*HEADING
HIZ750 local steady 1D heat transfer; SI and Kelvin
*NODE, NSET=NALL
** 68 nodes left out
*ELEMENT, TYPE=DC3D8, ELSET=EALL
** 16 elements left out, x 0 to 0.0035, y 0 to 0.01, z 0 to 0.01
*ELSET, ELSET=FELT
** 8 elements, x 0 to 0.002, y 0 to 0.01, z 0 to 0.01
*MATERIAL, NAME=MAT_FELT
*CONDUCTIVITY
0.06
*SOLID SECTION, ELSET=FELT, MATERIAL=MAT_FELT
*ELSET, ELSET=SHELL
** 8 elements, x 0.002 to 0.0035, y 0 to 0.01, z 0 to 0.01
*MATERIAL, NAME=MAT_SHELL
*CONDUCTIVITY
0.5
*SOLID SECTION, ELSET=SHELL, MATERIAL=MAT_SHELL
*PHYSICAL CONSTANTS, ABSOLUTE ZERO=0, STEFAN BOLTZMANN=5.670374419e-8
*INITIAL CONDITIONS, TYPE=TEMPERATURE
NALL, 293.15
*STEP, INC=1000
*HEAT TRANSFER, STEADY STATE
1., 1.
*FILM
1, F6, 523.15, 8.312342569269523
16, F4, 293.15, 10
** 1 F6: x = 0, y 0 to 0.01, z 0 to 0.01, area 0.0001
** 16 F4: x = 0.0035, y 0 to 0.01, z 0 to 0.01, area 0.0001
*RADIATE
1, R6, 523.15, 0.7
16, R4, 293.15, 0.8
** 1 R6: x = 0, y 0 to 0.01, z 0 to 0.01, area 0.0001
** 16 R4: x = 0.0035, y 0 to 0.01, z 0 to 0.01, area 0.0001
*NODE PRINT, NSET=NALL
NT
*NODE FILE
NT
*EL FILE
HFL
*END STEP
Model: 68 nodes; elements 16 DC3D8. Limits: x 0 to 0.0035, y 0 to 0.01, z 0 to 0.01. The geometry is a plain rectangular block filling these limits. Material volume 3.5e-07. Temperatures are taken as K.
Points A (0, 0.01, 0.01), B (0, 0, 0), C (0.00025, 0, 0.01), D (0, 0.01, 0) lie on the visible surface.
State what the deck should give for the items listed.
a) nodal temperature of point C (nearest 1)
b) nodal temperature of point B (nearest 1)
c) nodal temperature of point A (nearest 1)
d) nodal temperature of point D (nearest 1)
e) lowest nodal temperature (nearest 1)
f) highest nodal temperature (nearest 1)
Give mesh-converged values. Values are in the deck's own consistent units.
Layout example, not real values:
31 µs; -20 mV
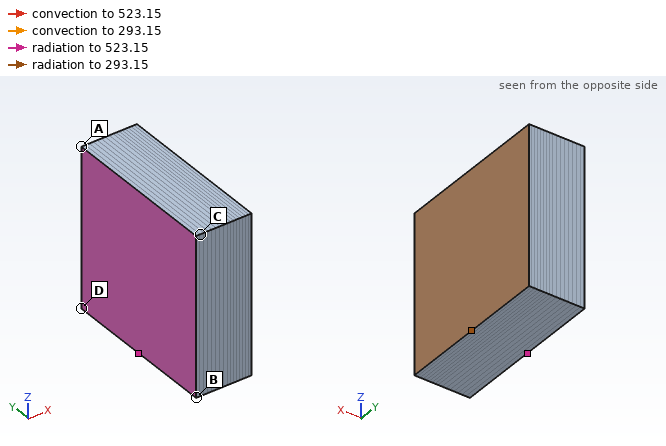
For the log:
451 K; 458 K; 458 K; 458 K; 394 K; 458 K
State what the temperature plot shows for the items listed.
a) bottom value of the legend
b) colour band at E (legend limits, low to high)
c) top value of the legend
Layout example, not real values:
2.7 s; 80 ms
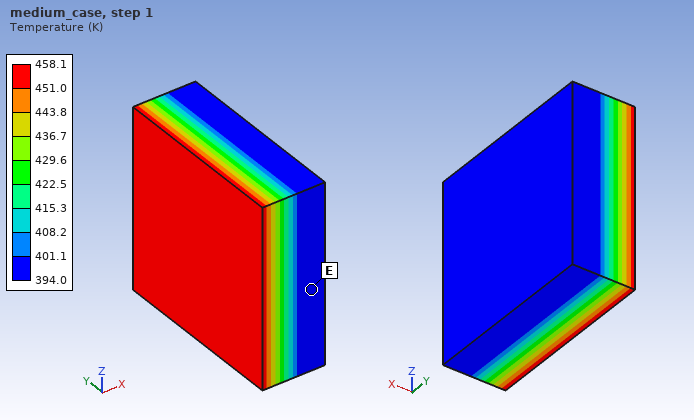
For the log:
394.0 K; 394.0 to 401.1 K; 458.1 K
